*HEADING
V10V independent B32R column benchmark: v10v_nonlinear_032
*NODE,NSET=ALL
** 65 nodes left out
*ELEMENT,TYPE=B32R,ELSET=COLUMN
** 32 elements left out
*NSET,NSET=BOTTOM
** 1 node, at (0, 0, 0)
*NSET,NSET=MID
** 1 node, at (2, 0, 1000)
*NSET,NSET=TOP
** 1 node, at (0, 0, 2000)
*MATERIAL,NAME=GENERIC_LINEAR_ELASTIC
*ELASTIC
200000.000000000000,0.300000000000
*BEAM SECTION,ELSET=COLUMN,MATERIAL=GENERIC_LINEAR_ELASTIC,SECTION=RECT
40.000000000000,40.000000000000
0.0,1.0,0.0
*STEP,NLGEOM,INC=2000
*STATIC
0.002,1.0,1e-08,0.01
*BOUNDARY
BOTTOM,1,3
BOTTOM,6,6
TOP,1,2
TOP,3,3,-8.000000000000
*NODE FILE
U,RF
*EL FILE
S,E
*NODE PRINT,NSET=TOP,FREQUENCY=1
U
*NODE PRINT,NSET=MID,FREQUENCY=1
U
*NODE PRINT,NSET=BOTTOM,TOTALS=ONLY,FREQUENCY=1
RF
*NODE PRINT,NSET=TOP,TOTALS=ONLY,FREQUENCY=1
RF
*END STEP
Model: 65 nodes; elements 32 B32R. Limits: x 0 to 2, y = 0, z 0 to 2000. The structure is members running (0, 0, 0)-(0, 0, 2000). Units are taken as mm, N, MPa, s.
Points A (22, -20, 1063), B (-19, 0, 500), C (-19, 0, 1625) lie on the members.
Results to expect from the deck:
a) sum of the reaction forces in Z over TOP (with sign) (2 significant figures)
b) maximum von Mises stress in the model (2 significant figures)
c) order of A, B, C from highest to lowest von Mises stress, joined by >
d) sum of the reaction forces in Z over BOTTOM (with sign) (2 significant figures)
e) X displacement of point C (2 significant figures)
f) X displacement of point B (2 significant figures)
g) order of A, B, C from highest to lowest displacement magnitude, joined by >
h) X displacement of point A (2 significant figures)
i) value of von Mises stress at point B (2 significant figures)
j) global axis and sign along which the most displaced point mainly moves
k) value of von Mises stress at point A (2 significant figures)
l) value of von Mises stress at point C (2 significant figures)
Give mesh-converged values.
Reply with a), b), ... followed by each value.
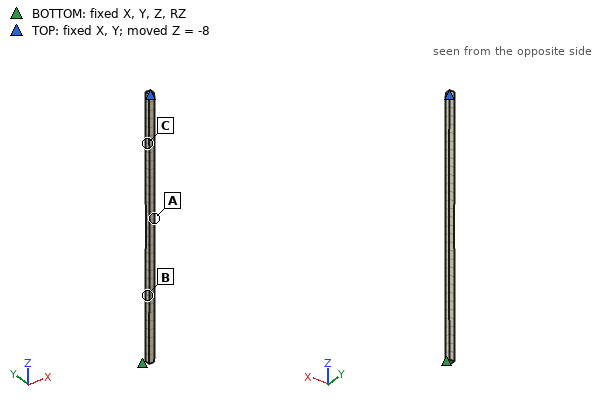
a) -1.0e+05 N
b) 800 MPa
c) A > B > C
d) 1.0e+05 N
e) 42 mm
f) 53 mm
g) A > B > C
h) 75 mm
i) 590 MPa
j) +X
k) 670 MPa
l) 470 MPa
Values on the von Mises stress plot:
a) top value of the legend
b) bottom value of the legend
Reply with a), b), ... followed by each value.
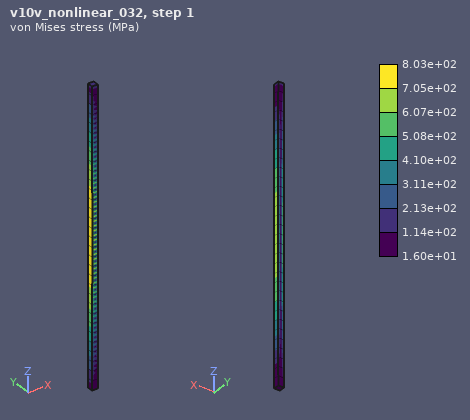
a) 8.03e+02 MPa
b) 1.60e+01 MPa
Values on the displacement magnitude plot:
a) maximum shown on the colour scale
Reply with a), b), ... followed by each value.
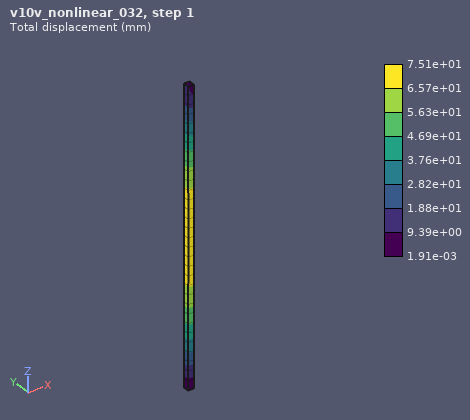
a) 7.51e+01 mm
